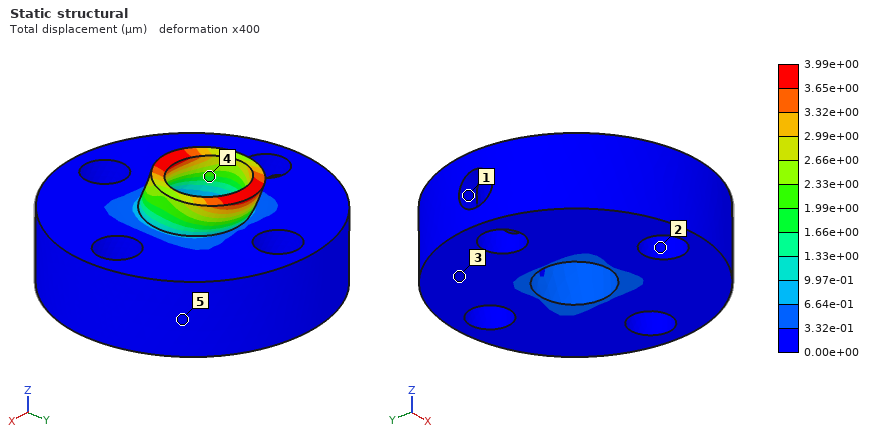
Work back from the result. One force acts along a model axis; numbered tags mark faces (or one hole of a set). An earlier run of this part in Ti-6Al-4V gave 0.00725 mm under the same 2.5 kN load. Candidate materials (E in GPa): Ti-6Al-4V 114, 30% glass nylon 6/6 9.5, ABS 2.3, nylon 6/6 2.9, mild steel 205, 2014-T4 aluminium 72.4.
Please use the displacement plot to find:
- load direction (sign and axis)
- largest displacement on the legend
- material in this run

+Y
3.99e+00 µm
mild steel
